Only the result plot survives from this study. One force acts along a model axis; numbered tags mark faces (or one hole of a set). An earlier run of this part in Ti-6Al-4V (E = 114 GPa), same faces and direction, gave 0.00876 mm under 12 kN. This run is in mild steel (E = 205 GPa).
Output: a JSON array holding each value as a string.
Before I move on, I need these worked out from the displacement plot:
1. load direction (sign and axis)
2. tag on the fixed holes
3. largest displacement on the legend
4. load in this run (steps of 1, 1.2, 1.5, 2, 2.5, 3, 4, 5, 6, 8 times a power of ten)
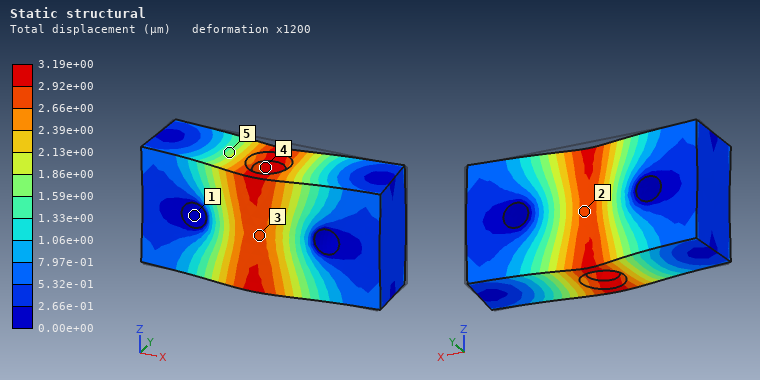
["-Y", "1", "3.19e+00 µm", "8 kN"]
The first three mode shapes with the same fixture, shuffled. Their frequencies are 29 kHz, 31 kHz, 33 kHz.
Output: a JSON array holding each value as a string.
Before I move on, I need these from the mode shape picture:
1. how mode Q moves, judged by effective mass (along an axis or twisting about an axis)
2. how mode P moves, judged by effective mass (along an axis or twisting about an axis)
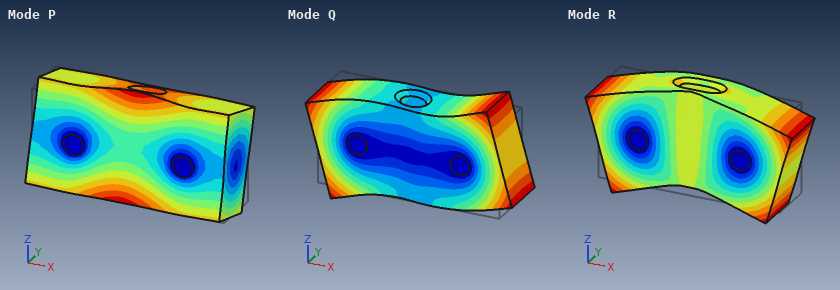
["twisting about Y", "twisting about X"]
